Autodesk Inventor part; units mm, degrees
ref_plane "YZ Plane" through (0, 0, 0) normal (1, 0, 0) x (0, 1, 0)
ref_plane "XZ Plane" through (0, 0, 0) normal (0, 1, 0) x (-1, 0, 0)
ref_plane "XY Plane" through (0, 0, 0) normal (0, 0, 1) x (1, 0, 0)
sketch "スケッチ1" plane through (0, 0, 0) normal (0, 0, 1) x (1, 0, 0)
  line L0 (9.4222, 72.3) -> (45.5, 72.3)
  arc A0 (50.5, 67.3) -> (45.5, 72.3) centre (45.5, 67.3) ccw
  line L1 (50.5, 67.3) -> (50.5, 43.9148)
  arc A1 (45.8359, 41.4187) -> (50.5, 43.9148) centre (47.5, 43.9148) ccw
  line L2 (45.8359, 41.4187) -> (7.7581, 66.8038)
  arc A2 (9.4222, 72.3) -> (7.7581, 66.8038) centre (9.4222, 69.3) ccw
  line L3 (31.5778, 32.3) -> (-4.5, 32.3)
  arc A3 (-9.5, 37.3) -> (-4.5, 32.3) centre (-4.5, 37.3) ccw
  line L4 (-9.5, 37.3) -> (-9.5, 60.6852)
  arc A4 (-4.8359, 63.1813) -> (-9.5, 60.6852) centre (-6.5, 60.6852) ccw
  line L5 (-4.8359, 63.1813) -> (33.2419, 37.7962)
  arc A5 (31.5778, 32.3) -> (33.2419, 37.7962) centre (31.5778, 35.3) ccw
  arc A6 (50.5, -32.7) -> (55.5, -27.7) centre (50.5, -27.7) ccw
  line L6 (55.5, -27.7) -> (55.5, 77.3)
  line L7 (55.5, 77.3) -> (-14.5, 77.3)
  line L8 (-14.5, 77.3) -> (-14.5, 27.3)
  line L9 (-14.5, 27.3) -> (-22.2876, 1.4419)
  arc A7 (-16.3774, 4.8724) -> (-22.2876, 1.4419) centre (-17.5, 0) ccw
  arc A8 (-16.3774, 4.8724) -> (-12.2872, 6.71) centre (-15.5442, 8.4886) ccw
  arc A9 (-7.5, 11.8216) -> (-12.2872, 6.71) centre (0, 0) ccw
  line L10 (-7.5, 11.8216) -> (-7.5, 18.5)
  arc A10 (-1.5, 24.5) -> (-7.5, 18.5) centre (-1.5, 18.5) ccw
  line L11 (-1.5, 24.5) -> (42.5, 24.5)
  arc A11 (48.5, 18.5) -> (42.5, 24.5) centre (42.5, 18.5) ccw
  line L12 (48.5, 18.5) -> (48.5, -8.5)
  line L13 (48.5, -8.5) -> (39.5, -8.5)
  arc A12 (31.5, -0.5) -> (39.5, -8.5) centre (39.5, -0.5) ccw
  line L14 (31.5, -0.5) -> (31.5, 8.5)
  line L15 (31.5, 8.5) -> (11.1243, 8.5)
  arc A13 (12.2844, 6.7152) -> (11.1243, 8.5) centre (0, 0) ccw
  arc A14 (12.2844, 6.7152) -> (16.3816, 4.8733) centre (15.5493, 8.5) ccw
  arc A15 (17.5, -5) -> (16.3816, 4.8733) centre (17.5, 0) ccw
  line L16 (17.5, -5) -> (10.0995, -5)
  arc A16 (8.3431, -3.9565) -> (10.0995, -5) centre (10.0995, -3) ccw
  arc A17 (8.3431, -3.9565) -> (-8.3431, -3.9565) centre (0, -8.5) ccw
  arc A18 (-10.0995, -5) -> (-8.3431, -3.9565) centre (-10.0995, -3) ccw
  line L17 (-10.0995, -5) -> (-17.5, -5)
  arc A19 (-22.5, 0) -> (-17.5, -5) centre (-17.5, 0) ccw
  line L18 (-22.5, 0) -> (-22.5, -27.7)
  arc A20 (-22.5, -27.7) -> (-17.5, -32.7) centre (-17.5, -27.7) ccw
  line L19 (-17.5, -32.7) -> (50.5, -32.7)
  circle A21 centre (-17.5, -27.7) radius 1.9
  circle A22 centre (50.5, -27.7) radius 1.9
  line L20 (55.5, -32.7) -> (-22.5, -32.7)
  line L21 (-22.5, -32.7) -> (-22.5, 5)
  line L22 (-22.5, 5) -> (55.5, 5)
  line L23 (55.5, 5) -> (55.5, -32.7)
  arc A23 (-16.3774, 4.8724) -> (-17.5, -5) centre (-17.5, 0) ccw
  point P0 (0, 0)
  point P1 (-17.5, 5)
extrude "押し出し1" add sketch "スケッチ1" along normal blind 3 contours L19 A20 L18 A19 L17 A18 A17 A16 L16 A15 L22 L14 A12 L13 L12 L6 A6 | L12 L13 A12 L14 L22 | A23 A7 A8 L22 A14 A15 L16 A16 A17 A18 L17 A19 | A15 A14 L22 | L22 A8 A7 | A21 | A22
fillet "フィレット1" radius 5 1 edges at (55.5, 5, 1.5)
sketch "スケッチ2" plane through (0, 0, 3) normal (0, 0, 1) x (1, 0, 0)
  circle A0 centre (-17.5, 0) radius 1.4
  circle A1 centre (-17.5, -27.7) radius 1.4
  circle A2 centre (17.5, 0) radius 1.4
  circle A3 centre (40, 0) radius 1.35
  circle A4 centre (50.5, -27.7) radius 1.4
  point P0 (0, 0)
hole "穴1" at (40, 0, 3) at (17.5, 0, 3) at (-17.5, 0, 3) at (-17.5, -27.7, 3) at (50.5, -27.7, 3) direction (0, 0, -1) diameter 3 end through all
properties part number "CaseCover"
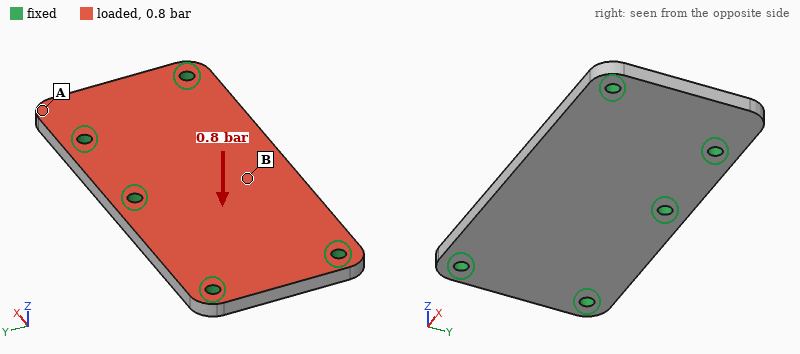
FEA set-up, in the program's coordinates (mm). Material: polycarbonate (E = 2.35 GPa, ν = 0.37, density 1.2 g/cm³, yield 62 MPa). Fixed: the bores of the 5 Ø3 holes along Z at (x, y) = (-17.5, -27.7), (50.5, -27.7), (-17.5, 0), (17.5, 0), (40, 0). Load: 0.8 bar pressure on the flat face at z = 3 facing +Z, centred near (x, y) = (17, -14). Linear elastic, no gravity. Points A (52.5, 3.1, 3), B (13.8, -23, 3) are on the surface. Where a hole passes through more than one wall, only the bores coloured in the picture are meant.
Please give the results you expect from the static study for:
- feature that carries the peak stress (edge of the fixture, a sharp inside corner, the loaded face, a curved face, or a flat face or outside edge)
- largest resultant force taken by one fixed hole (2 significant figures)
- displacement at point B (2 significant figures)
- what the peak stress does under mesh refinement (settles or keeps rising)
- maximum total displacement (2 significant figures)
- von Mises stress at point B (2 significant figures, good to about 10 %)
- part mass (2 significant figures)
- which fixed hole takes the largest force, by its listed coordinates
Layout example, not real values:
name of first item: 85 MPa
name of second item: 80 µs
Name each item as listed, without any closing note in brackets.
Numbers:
feature that carries the peak stress: edge of the fixture
largest resultant force taken by one fixed hole: 69 N
displacement at point B: 0.43 mm
what the peak stress does under mesh refinement: keeps rising
maximum total displacement: 0.63 mm
von Mises stress at point B: 4.4 MPa
part mass: 10 g
which fixed hole takes the largest force, by its listed coordinates: (17.5, 0)
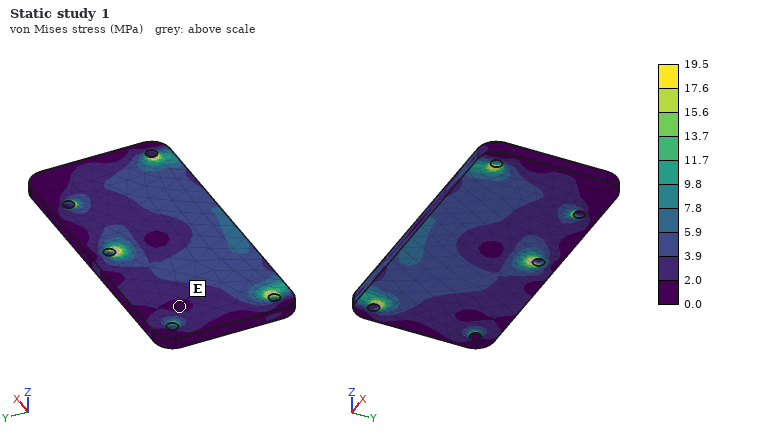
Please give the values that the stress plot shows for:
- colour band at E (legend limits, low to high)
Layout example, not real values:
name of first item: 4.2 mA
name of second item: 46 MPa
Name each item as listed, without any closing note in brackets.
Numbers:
colour band at E: 0.0 to 2.0 MPa
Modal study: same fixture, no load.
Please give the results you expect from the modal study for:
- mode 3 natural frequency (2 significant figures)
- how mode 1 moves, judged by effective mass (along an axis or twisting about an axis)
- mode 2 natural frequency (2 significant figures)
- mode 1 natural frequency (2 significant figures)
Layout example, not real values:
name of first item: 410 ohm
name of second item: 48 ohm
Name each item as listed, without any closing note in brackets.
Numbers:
mode 3 natural frequency: 3300 Hz
how mode 1 moves, judged by effective mass: along Z
mode 2 natural frequency: 2700 Hz
mode 1 natural frequency: 1300 Hz
